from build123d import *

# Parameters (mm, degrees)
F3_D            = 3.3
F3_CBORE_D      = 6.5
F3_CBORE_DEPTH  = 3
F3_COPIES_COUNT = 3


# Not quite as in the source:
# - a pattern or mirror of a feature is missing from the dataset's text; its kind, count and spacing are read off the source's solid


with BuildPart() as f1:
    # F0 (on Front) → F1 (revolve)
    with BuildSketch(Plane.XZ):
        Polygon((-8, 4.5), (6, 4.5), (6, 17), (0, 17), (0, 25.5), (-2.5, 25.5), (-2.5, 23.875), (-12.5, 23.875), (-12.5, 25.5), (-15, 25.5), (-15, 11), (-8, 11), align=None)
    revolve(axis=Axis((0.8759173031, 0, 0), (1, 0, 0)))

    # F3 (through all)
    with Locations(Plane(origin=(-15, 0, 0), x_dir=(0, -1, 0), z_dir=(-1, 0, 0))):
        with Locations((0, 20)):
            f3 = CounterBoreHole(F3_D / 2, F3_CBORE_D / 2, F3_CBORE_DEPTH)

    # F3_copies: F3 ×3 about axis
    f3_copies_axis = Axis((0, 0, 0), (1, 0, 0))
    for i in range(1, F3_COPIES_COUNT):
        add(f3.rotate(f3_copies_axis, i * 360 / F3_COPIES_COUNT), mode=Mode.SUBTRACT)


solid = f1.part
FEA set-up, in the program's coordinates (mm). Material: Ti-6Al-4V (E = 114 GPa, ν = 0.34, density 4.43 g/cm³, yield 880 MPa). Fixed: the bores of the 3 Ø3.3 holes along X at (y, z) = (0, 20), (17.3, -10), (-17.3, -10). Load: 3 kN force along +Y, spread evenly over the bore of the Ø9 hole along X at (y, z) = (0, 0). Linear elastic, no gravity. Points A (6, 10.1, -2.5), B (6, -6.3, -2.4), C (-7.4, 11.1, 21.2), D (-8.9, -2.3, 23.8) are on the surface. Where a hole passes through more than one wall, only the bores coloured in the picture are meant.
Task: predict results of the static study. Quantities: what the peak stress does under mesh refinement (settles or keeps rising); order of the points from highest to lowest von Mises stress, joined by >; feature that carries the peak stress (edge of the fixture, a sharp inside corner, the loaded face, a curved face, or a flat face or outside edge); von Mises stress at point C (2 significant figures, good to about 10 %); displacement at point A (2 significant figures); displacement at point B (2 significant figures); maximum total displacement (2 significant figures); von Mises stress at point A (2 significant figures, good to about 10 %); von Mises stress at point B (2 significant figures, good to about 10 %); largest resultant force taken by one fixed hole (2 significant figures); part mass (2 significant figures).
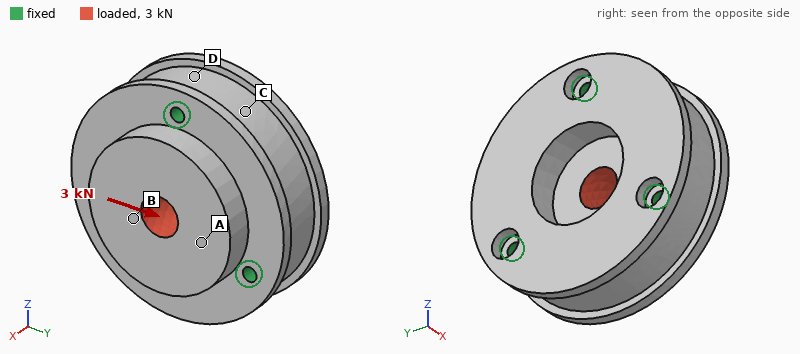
keeps rising
B > A > C > D
edge of the fixture
3.2 MPa
1.4 µm
1.5 µm
1.9 µm
6.5 MPa
9.2 MPa
1.1 kN
130 g
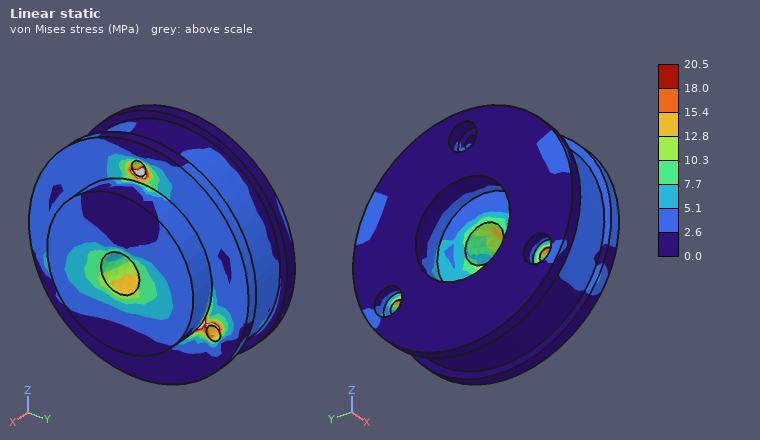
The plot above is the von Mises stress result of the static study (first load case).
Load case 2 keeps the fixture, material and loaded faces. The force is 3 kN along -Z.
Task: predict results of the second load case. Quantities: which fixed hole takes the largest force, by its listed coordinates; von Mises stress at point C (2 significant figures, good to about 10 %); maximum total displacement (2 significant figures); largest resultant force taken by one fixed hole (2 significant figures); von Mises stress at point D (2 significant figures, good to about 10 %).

(0, 20)
2.4 MPa
2.1 µm
1.1 kN
4.0 MPa
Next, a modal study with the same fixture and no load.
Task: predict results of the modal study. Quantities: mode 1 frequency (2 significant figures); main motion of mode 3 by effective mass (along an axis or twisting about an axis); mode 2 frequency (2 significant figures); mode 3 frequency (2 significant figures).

22 kHz
along X
22 kHz
24 kHz
